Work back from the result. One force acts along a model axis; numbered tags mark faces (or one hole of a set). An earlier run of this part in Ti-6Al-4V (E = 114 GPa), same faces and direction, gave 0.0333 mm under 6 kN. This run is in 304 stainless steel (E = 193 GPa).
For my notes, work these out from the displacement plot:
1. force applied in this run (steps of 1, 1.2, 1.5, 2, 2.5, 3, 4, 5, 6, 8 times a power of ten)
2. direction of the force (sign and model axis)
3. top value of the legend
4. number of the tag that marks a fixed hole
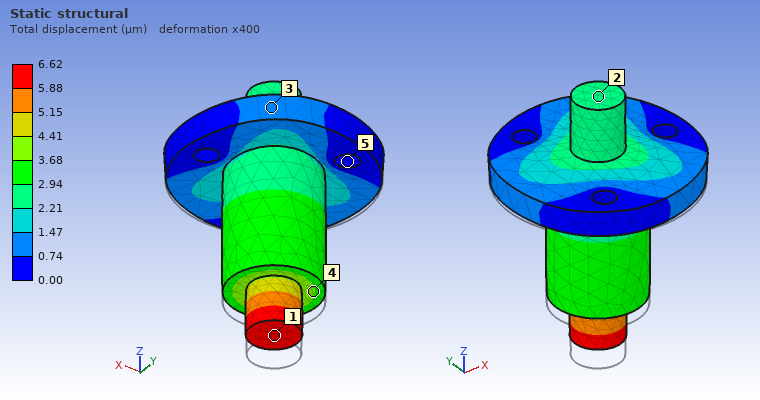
2 kN
+Z
6.62 µm
5
